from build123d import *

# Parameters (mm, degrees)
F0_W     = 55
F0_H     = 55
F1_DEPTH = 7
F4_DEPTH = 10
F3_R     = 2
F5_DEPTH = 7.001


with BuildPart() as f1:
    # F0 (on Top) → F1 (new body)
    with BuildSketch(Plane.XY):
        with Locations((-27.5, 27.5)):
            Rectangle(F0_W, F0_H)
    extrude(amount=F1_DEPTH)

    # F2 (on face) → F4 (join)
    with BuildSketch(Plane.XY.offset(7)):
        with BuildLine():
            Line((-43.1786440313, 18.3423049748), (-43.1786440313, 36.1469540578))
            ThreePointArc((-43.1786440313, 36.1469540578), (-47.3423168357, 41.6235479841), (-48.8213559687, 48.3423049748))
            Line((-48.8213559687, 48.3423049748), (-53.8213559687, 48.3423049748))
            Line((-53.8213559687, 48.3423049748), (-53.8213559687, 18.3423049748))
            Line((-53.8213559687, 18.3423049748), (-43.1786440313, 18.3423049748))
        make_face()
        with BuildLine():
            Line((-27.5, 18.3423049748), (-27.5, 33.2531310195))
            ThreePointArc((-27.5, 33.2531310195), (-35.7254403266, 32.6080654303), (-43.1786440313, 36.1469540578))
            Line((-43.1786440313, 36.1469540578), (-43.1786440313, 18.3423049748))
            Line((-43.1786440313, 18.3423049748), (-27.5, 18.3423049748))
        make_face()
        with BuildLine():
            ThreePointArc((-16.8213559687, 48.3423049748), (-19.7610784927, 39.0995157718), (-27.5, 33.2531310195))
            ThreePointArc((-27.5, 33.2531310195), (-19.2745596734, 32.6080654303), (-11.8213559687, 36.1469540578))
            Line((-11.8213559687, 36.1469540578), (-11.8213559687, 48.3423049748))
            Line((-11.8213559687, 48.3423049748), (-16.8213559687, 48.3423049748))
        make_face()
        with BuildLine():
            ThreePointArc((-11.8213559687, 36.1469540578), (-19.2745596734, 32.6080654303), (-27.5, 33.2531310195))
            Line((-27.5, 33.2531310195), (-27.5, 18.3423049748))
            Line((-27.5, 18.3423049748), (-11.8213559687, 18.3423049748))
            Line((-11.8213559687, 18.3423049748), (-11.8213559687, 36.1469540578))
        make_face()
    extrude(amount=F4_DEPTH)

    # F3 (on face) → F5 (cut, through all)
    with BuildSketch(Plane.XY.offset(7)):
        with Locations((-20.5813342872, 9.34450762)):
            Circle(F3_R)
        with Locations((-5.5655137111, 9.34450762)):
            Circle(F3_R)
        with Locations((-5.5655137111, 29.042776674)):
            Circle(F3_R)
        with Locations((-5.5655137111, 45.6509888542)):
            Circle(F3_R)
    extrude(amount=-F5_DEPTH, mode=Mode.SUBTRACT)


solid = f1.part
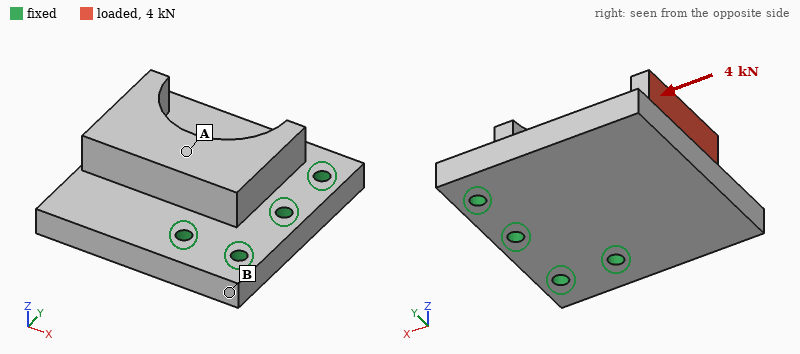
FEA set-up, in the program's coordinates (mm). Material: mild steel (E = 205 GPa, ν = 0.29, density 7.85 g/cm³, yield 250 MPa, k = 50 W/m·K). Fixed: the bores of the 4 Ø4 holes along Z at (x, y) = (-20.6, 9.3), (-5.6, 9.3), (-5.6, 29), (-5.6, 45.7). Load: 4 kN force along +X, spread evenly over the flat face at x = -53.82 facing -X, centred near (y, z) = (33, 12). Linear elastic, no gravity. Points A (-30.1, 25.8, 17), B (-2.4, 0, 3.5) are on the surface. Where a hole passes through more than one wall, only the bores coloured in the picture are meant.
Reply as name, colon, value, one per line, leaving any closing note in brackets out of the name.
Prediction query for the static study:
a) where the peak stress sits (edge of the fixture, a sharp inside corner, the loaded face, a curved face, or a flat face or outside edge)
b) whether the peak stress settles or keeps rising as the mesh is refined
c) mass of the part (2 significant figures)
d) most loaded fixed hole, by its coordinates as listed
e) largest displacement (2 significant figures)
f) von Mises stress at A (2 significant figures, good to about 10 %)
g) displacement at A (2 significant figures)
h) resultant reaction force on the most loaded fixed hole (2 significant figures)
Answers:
where the peak stress sits: edge of the fixture
whether the peak stress settles or keeps rising as the mesh is refined: keeps rising
mass of the part: 230 g
most loaded fixed hole, by its coordinates as listed: (-5.6, 29)
largest displacement: 43 µm
von Mises stress at A: 33 MPa
displacement at A: 15 µm
resultant reaction force on the most loaded fixed hole: 2.0 kN
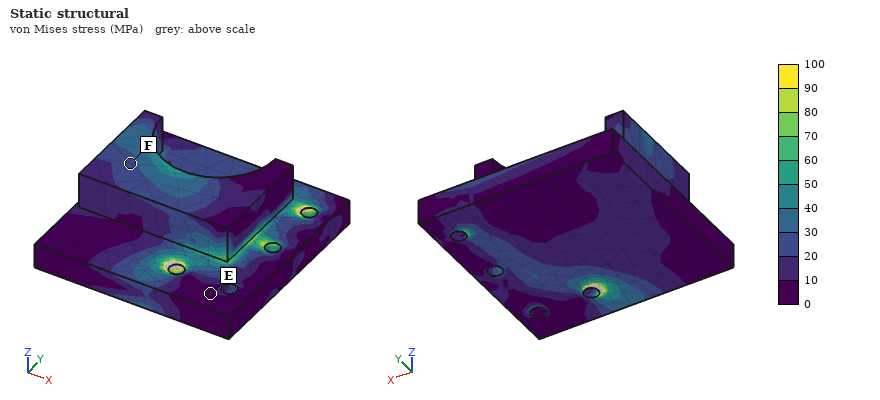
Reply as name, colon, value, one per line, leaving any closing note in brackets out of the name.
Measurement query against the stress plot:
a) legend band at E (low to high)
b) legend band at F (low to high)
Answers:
legend band at E: 0 to 10 MPa
legend band at F: 20 to 30 MPa
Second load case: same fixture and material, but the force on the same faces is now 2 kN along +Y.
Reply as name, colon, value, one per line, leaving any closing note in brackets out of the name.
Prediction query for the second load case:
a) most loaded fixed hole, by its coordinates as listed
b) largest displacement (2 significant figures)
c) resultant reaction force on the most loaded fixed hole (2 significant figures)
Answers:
most loaded fixed hole, by its coordinates as listed: (-20.6, 9.3)
largest displacement: 16 µm
resultant reaction force on the most loaded fixed hole: 2.2 kN
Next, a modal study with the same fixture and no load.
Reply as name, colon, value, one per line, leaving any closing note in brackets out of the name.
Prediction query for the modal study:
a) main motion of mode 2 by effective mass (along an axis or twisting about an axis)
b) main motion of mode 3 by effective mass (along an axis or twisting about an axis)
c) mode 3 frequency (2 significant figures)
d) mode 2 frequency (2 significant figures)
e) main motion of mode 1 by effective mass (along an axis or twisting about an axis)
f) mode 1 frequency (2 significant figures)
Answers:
main motion of mode 2 by effective mass: twisting about X
main motion of mode 3 by effective mass: along Y
mode 3 frequency: 11 kHz
mode 2 frequency: 8600 Hz
main motion of mode 1 by effective mass: along Z
mode 1 frequency: 3200 Hz
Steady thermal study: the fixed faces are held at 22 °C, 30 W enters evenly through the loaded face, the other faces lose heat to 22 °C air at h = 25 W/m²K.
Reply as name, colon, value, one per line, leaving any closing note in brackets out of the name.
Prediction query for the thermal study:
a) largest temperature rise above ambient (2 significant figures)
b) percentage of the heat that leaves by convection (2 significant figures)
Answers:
largest temperature rise above ambient: 65 K
percentage of the heat that leaves by convection: 15 %
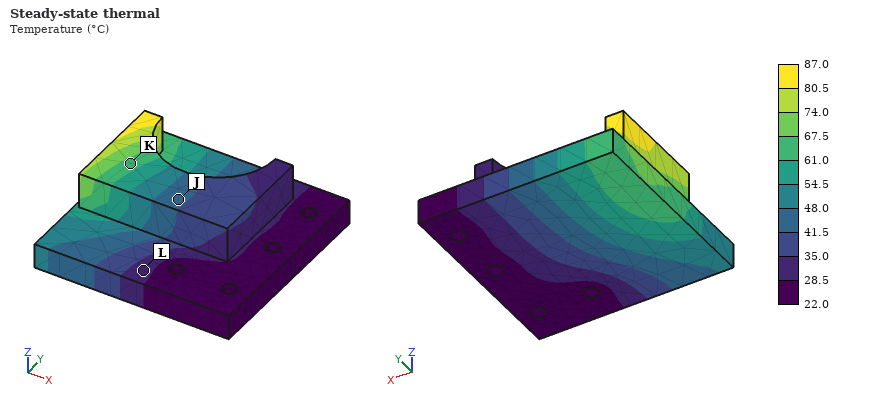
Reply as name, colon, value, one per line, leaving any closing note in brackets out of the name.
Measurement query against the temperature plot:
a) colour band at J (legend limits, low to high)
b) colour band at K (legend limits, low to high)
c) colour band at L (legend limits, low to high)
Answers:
colour band at J: 41.5 to 48.0 °C
colour band at K: 61.0 to 67.5 °C
colour band at L: 28.5 to 35.0 °C
